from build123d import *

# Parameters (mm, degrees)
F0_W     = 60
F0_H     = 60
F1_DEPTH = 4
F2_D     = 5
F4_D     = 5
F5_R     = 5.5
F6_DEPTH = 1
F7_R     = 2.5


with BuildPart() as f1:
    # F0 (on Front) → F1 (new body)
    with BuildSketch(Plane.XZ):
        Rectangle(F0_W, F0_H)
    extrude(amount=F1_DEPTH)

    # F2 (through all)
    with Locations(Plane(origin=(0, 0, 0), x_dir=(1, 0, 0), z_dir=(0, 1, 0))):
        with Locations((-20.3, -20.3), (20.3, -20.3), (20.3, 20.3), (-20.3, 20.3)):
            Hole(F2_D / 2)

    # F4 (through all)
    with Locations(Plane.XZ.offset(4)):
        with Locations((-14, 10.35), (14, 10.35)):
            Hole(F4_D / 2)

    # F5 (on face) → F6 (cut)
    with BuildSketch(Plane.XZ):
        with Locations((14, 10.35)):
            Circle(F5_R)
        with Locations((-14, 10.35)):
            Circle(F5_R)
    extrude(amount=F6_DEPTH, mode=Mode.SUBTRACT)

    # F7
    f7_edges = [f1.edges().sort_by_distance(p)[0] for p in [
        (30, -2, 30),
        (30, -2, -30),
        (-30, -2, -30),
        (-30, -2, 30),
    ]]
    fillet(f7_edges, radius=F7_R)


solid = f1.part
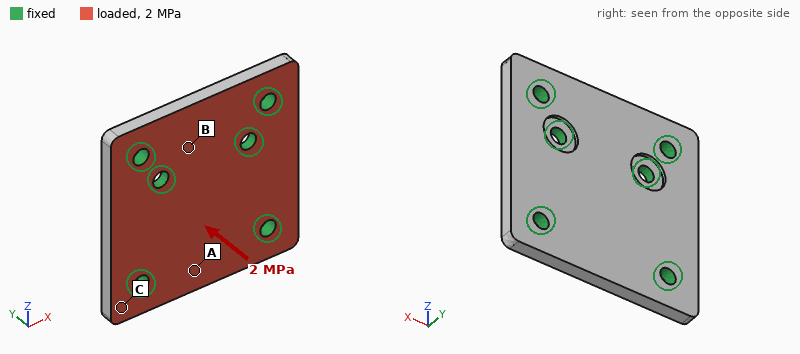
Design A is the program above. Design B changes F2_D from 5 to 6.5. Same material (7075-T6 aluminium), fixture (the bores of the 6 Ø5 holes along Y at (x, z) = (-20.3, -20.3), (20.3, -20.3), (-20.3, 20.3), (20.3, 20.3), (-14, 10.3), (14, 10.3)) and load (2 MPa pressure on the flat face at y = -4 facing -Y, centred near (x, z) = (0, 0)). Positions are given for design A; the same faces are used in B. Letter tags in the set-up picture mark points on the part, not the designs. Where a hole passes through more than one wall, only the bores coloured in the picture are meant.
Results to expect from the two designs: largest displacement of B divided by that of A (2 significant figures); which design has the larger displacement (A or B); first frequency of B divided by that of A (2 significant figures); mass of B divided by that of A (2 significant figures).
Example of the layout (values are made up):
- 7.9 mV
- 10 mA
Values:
- 0.82
- A
- 1.1
- 0.98
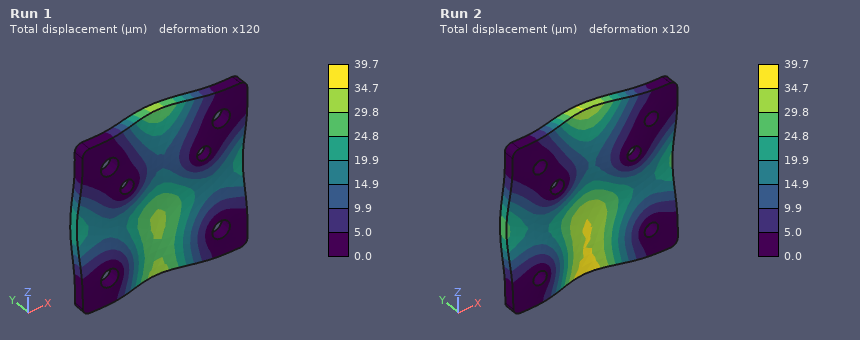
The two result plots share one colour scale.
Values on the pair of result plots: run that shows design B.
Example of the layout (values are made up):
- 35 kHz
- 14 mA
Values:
- Run 1
